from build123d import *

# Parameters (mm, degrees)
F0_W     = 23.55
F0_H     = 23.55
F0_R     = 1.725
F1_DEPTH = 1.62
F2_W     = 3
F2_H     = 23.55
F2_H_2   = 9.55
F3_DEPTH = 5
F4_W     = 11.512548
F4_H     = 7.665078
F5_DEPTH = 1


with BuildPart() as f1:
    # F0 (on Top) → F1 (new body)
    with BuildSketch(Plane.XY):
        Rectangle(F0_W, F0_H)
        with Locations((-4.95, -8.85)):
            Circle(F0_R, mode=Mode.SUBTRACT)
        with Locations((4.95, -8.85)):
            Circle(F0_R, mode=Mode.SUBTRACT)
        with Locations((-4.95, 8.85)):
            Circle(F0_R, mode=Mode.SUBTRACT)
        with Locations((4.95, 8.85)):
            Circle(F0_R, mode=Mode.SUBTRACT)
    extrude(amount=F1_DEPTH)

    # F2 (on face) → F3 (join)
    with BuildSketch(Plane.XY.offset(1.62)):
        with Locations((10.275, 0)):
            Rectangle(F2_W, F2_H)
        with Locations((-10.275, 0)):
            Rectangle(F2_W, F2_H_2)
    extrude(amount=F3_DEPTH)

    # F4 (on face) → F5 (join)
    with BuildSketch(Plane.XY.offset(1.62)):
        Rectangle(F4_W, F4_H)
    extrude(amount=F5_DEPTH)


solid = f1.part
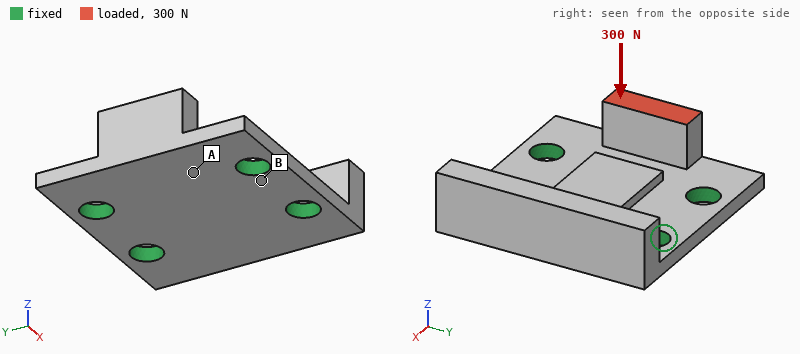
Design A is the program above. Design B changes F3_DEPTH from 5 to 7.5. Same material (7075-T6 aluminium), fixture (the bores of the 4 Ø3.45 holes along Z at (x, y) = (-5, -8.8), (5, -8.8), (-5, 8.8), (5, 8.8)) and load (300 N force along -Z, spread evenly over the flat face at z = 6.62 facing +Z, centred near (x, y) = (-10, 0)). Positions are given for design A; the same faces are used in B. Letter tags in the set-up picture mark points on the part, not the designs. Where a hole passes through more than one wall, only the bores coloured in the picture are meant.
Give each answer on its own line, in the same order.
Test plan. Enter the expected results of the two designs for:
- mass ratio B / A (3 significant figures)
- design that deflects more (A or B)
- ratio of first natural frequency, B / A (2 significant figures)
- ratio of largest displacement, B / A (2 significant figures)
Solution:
1.17
B
0.68
1.2
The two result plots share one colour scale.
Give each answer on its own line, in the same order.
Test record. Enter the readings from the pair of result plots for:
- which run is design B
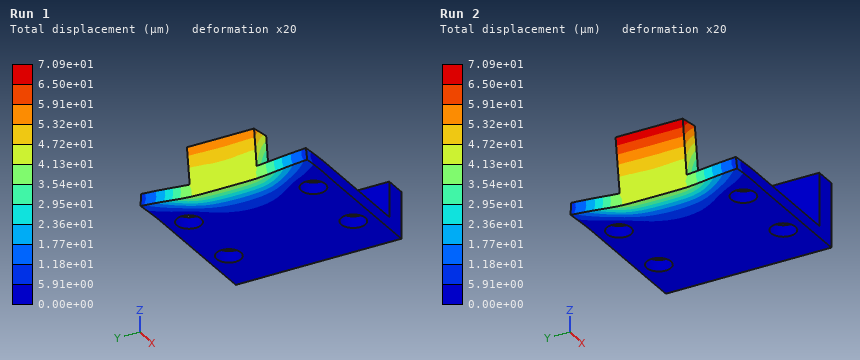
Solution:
Run 2
